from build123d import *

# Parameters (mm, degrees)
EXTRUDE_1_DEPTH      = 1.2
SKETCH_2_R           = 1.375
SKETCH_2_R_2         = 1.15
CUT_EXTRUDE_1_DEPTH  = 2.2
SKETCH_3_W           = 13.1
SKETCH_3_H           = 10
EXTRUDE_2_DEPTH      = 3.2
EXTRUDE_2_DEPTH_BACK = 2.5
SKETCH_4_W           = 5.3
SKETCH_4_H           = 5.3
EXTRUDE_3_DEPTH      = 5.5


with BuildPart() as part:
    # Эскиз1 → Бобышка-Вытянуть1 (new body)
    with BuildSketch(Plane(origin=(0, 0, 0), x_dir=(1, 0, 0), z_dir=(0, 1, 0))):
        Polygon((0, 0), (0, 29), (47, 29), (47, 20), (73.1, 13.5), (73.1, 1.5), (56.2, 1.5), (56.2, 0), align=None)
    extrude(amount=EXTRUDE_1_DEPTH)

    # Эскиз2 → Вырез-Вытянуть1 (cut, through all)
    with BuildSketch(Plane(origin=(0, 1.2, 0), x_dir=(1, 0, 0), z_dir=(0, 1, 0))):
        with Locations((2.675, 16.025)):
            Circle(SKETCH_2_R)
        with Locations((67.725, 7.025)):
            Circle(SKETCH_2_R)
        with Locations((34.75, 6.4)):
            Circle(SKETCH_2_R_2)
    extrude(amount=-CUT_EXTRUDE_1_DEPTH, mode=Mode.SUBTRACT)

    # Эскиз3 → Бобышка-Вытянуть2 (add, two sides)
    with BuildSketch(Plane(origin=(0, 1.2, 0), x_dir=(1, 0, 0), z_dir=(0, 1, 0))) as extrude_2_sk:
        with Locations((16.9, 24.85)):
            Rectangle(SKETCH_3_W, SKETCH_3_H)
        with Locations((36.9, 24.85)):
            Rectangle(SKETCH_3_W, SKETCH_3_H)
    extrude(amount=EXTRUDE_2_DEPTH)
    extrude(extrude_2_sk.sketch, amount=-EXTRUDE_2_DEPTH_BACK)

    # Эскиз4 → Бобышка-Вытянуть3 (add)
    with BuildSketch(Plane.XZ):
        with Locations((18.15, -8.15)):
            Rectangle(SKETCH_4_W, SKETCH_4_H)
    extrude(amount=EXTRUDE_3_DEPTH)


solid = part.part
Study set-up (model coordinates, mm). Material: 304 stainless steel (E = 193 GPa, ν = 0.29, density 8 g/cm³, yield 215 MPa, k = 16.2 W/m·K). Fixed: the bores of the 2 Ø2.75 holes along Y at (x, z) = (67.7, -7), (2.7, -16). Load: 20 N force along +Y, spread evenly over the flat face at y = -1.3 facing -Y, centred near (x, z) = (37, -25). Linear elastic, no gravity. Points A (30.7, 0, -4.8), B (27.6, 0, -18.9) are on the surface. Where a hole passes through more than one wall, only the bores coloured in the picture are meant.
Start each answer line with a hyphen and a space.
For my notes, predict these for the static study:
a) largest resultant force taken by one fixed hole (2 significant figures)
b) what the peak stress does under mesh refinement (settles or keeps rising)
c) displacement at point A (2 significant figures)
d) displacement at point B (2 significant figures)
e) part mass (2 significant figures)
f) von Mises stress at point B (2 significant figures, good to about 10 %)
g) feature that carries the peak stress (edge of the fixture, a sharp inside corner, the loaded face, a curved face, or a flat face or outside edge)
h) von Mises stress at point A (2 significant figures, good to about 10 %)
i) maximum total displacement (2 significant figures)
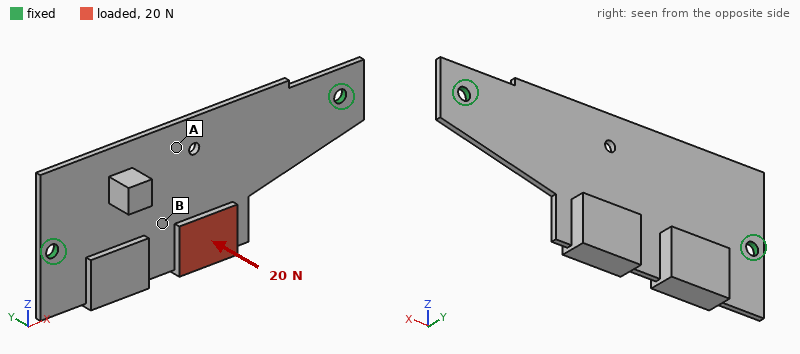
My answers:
- 10 N
- keeps rising
- 15 µm
- 43 µm
- 28 g
- 16 MPa
- edge of the fixture
- 8.1 MPa
- 86 µm
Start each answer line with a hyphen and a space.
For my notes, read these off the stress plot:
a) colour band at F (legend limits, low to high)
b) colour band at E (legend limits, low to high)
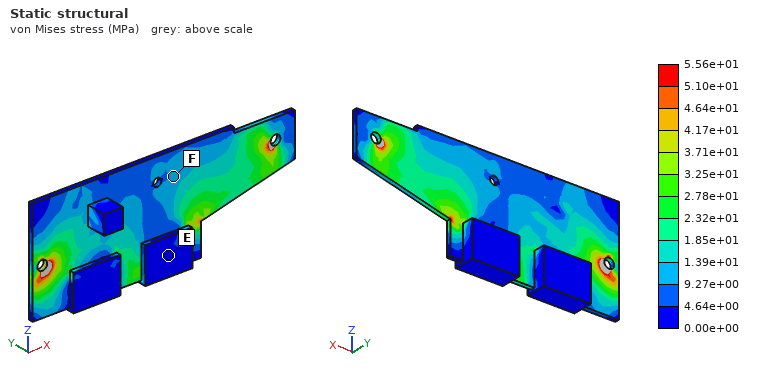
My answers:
- 9.27e+00 to 1.39e+01 MPa
- 0.00e+00 to 4.64e+00 MPa
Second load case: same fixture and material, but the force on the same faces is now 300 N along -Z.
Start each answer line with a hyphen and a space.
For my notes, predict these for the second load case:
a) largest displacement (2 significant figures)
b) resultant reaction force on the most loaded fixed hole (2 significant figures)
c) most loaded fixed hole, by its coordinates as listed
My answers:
- 0.12 mm
- 170 N
- (67.7, -7)
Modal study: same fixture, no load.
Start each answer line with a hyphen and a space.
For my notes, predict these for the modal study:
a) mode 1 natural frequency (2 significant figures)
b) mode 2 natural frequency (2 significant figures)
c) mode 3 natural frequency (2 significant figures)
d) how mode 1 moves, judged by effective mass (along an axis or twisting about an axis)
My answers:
- 850 Hz
- 1500 Hz
- 3000 Hz
- along Y
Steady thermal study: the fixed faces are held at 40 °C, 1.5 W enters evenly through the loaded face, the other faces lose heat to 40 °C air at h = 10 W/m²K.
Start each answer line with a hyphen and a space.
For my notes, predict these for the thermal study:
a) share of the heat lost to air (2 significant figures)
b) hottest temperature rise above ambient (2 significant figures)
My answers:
- 51 %
- 44 K
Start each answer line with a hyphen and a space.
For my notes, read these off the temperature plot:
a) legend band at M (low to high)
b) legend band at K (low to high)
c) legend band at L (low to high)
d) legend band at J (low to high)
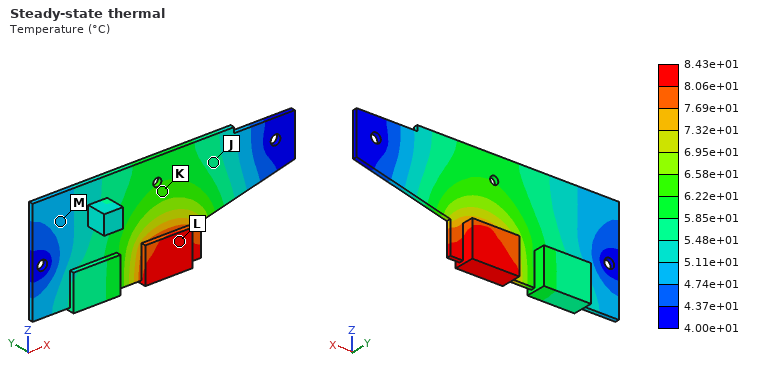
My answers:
- 4.74e+01 to 5.11e+01 °C
- 6.22e+01 to 6.58e+01 °C
- 8.06e+01 to 8.43e+01 °C
- 5.48e+01 to 5.85e+01 °C
